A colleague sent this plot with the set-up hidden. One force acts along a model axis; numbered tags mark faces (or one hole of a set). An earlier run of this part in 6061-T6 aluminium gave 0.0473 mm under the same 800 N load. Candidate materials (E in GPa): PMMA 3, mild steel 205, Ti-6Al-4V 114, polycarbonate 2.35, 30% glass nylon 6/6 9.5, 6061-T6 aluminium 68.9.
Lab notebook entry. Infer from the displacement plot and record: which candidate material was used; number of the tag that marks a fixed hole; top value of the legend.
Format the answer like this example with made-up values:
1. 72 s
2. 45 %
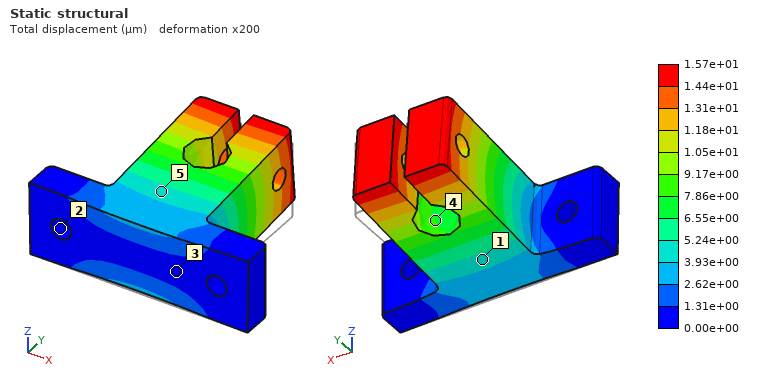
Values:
1. mild steel
2. 2
3. 1.57e+01 µm
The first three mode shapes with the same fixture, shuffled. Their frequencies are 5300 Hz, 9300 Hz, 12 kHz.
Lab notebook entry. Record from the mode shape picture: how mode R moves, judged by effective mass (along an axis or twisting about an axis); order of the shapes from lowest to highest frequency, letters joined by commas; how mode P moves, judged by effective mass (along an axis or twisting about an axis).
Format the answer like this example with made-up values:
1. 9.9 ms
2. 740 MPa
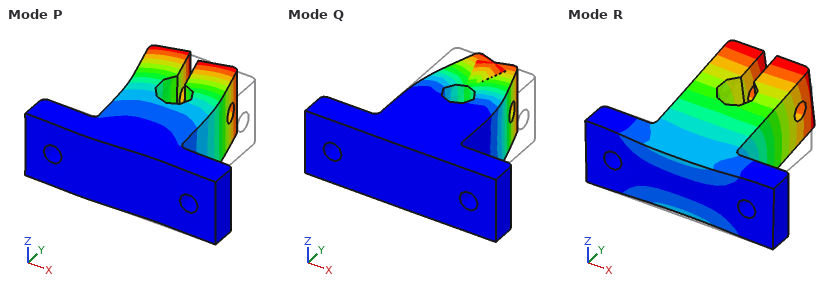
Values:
1. along Z
2. R, P, Q
3. along X
